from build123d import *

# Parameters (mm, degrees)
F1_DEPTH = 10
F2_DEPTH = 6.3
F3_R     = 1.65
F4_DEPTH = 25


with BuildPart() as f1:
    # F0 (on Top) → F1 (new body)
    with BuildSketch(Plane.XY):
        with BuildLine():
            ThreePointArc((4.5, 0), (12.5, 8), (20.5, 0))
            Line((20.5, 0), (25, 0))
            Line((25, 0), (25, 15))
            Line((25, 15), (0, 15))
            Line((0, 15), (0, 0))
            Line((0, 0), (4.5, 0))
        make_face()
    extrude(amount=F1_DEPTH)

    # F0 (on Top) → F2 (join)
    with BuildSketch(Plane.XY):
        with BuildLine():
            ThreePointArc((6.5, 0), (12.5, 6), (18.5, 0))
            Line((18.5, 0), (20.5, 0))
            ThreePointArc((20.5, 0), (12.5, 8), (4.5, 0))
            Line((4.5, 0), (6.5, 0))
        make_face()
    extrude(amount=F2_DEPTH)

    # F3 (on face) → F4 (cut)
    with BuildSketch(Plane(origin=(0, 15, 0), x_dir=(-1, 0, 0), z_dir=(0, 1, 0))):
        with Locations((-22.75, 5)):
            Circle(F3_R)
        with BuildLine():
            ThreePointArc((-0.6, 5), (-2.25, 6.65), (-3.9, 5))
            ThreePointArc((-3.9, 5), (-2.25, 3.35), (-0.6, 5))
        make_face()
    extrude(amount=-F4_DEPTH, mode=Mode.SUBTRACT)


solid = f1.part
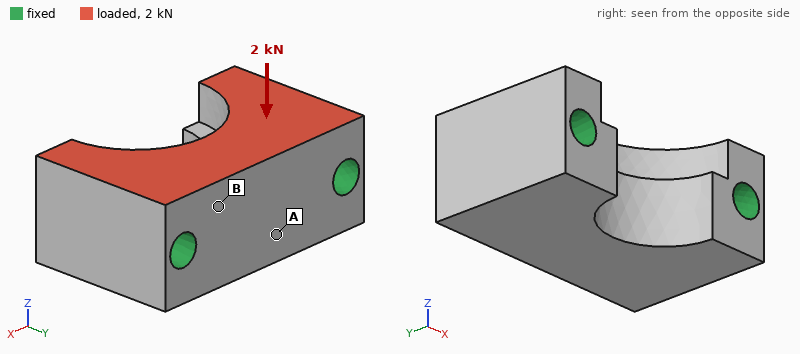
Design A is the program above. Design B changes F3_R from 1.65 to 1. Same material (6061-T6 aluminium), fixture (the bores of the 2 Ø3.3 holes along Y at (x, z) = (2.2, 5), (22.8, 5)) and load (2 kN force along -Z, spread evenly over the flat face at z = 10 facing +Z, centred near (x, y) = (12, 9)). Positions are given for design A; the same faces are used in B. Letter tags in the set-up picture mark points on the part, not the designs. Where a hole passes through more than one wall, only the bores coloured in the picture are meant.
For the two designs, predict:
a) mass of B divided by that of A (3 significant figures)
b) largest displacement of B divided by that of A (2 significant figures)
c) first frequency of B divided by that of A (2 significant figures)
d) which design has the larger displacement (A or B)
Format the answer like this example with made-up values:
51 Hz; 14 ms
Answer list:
1.03; 1.1; 0.91; B
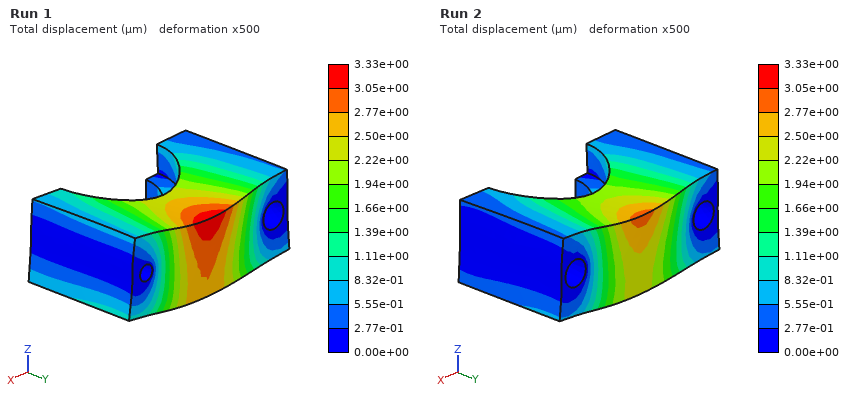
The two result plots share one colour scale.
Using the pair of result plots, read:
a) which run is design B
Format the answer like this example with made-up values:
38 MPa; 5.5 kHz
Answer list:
Run 1
